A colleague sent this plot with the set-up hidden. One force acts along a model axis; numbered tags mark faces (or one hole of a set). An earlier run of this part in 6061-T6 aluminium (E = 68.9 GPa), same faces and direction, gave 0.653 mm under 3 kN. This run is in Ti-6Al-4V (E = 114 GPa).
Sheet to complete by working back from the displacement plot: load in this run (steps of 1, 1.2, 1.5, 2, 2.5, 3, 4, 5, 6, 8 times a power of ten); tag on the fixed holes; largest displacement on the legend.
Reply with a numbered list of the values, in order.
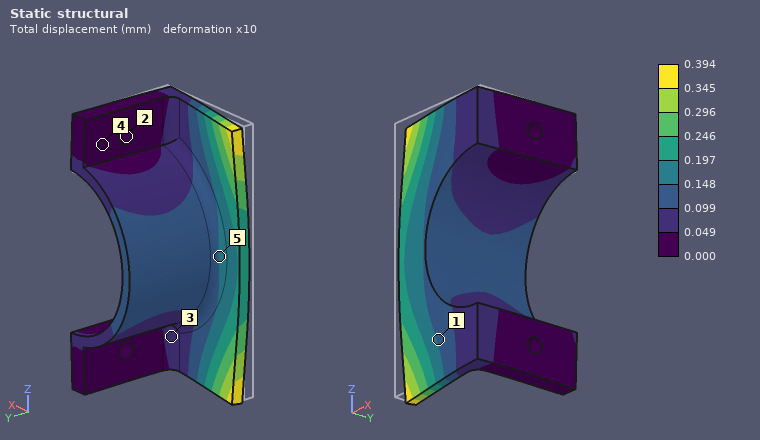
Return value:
1. 3 kN
2. 2
3. 0.394 mm
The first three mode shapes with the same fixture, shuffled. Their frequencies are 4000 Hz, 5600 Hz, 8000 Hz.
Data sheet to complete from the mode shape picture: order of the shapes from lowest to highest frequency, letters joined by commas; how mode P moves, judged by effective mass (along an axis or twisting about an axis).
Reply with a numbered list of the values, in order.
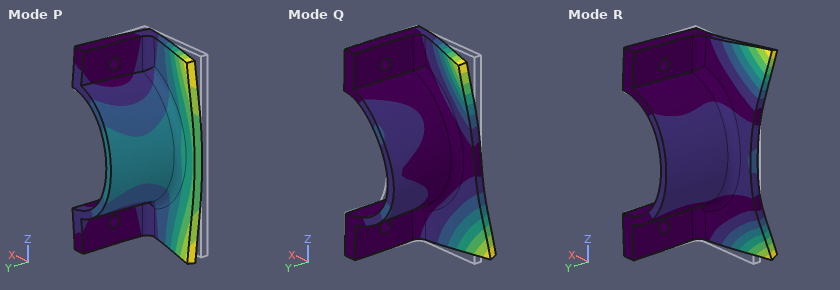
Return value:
1. P, Q, R
2. along Y
